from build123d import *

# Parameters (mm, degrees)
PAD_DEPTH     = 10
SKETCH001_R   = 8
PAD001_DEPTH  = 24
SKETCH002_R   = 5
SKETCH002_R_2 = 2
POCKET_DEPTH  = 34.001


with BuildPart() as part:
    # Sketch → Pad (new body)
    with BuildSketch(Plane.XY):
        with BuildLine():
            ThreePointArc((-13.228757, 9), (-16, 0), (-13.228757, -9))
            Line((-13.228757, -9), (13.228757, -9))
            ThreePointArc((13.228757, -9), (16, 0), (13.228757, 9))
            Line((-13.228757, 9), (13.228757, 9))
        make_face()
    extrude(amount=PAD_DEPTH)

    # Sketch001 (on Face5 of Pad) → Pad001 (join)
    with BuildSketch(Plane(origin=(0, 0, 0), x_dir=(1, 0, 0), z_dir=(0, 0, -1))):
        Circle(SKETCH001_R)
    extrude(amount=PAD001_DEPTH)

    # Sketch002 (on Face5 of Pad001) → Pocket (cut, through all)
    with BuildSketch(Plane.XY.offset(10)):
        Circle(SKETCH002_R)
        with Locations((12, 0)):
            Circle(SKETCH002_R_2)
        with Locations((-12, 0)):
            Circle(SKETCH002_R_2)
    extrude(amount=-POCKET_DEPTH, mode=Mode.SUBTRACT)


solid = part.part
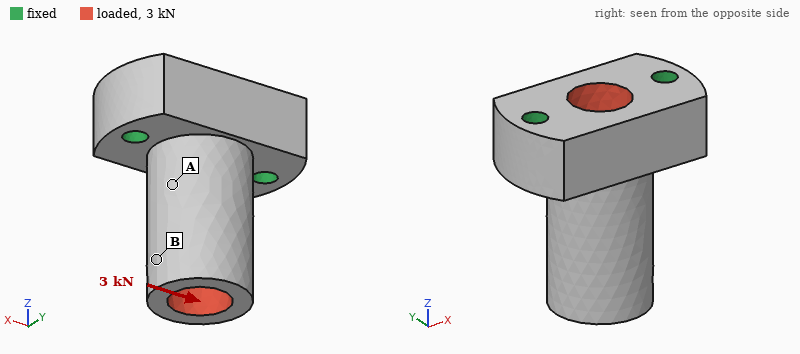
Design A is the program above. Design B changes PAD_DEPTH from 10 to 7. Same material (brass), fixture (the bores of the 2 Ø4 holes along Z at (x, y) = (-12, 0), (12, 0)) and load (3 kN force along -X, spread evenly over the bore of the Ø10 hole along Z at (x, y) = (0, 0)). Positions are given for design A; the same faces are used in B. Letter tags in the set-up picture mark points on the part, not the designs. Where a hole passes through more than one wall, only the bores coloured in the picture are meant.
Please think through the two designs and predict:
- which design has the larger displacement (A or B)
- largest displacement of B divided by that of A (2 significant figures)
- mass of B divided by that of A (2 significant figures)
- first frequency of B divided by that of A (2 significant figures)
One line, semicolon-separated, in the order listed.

B; 1.2; 0.82; 0.83
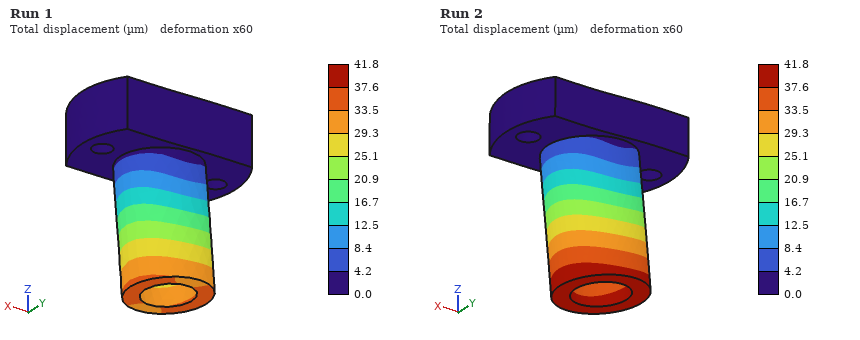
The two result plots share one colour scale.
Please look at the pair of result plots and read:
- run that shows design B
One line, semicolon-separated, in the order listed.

Run 2
